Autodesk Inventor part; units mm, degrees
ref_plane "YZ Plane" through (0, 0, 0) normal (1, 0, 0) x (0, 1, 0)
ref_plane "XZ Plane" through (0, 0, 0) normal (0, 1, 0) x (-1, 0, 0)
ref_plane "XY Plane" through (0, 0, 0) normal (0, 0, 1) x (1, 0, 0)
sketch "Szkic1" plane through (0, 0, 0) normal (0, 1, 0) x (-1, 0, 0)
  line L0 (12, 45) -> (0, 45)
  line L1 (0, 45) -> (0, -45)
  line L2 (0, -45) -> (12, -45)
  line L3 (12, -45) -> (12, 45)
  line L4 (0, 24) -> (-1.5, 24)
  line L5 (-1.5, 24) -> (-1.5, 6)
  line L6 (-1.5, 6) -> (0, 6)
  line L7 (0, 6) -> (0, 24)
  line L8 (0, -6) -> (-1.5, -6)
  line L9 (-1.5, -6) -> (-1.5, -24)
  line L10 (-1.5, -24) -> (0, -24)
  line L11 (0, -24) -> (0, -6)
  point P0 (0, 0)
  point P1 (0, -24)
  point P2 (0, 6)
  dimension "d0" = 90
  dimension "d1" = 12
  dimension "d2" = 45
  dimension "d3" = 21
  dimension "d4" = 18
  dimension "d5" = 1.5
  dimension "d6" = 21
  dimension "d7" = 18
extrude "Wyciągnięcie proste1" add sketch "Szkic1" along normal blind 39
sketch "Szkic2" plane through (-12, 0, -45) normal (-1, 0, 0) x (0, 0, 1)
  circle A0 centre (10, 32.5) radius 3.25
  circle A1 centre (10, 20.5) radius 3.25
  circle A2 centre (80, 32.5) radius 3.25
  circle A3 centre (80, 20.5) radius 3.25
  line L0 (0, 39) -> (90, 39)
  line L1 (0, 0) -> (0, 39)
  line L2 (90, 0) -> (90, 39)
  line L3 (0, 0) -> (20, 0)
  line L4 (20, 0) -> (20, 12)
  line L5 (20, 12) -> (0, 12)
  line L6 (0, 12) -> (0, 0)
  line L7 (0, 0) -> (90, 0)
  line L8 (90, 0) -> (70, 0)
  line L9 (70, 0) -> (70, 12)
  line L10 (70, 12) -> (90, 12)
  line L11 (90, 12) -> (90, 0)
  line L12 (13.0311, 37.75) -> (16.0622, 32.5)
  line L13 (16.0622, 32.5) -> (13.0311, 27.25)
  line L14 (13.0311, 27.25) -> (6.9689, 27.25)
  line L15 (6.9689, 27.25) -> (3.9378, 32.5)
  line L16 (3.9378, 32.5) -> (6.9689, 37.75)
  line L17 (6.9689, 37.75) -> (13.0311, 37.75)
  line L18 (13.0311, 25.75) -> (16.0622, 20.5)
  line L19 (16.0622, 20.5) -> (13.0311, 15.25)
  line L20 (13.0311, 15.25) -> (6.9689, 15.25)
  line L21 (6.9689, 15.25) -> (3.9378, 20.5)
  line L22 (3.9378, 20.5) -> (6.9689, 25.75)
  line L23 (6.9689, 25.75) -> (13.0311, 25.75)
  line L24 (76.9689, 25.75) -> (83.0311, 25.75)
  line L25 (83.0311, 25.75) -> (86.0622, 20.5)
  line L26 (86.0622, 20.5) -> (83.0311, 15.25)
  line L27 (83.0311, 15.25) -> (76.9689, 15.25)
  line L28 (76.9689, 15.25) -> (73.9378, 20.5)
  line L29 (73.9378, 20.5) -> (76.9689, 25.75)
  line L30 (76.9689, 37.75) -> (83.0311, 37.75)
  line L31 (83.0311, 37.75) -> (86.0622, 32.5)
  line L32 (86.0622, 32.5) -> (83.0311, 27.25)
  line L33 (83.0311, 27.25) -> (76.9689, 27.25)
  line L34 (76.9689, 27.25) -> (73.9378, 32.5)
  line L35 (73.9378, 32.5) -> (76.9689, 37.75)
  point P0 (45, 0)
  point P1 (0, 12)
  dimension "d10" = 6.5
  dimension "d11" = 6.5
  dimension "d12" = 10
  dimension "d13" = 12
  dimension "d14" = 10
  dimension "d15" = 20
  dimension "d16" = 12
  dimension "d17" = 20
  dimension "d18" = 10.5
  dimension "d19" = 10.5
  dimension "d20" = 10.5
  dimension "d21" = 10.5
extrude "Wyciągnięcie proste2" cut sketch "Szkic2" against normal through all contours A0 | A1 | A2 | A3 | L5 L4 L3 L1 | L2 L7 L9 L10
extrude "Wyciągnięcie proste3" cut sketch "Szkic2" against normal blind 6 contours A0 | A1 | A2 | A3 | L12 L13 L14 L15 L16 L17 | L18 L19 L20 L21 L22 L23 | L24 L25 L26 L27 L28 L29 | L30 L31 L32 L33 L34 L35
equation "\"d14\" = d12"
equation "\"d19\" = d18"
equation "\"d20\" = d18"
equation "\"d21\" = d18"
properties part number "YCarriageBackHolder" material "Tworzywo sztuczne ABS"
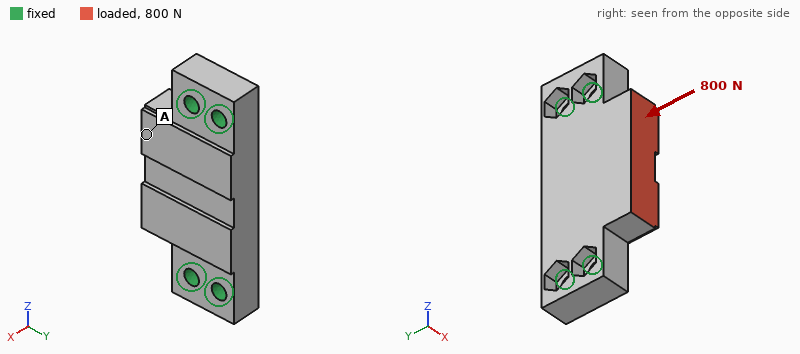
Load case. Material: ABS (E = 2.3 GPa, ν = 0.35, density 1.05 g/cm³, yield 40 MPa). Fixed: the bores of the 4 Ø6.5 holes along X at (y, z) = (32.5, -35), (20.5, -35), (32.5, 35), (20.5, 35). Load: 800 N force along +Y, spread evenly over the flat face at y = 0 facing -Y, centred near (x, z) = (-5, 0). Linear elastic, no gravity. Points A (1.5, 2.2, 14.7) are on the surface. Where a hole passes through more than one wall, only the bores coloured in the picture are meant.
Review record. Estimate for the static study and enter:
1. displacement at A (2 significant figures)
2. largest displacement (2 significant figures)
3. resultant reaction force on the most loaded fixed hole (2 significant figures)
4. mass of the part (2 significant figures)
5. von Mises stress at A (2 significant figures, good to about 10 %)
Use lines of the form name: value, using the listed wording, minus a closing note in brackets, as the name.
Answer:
displacement at A: 47 µm
largest displacement: 66 µm
resultant reaction force on the most loaded fixed hole: 280 N
mass of the part: 37 g
von Mises stress at A: 1.2 MPa
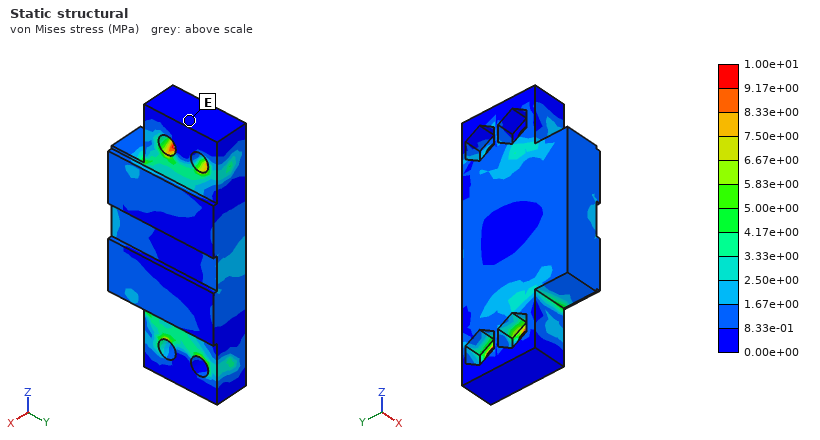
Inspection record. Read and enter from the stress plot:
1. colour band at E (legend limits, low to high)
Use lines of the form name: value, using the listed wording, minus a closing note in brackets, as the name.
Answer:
colour band at E: 0.00e+00 to 8.33e-01 MPa
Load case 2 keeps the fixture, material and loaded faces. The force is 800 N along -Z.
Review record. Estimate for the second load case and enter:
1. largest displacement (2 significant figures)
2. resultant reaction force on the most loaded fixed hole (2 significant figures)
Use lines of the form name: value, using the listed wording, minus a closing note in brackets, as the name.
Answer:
largest displacement: 74 µm
resultant reaction force on the most loaded fixed hole: 300 N
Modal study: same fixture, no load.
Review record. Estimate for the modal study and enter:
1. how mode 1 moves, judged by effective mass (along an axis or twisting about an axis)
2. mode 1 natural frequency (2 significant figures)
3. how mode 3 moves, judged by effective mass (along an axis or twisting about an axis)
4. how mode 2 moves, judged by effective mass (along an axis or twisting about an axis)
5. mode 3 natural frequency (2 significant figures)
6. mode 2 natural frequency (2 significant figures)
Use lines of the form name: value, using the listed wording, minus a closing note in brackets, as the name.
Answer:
how mode 1 moves, judged by effective mass: along X
mode 1 natural frequency: 2000 Hz
how mode 3 moves, judged by effective mass: along Y
how mode 2 moves, judged by effective mass: along X
mode 3 natural frequency: 4100 Hz
mode 2 natural frequency: 3200 Hz
